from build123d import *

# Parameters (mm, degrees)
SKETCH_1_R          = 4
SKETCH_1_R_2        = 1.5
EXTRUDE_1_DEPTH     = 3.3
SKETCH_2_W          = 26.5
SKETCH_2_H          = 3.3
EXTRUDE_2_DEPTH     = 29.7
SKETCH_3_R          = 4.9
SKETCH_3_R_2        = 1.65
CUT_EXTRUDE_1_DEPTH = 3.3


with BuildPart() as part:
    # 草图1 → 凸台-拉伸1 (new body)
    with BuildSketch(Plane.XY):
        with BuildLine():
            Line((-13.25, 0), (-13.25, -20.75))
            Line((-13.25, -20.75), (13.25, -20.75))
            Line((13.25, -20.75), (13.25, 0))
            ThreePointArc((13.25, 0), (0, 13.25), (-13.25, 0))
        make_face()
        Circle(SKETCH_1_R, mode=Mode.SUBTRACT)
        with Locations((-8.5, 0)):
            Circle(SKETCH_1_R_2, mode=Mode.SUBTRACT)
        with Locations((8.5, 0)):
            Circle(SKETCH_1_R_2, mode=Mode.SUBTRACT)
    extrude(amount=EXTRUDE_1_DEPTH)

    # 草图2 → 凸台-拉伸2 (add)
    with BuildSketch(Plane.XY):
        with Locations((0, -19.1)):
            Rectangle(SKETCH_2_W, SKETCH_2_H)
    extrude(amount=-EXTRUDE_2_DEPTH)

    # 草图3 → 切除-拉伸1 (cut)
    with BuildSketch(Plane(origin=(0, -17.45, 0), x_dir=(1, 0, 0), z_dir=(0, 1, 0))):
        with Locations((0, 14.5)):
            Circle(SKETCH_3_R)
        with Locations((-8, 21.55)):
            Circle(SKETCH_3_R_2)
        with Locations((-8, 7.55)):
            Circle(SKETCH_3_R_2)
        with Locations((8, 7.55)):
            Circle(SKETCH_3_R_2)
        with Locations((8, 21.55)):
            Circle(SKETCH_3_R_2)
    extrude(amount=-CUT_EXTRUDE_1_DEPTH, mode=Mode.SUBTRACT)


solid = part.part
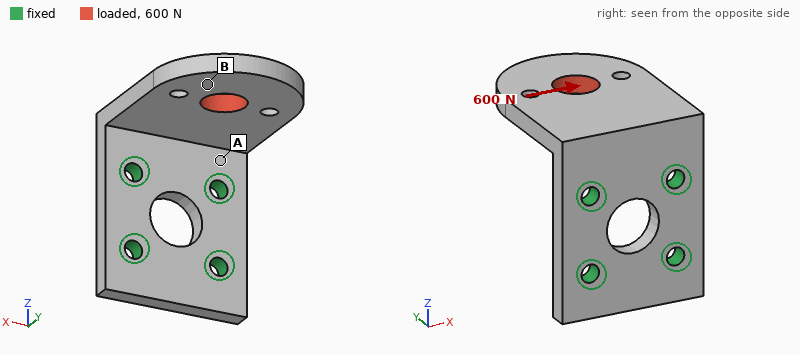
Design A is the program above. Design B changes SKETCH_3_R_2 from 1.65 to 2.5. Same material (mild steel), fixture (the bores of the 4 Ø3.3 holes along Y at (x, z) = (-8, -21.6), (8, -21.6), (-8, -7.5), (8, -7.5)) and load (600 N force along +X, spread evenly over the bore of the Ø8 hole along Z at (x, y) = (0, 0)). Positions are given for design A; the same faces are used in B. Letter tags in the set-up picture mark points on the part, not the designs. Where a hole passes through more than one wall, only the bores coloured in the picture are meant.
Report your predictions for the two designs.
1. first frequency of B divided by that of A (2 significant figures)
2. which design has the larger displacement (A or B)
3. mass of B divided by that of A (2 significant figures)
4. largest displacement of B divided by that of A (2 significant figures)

1.0
A
0.97
0.80
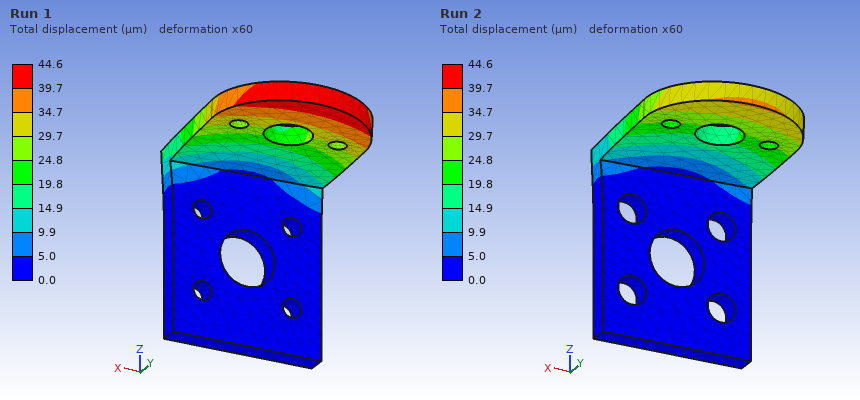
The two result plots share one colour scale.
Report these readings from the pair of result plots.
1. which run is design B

Run 2
